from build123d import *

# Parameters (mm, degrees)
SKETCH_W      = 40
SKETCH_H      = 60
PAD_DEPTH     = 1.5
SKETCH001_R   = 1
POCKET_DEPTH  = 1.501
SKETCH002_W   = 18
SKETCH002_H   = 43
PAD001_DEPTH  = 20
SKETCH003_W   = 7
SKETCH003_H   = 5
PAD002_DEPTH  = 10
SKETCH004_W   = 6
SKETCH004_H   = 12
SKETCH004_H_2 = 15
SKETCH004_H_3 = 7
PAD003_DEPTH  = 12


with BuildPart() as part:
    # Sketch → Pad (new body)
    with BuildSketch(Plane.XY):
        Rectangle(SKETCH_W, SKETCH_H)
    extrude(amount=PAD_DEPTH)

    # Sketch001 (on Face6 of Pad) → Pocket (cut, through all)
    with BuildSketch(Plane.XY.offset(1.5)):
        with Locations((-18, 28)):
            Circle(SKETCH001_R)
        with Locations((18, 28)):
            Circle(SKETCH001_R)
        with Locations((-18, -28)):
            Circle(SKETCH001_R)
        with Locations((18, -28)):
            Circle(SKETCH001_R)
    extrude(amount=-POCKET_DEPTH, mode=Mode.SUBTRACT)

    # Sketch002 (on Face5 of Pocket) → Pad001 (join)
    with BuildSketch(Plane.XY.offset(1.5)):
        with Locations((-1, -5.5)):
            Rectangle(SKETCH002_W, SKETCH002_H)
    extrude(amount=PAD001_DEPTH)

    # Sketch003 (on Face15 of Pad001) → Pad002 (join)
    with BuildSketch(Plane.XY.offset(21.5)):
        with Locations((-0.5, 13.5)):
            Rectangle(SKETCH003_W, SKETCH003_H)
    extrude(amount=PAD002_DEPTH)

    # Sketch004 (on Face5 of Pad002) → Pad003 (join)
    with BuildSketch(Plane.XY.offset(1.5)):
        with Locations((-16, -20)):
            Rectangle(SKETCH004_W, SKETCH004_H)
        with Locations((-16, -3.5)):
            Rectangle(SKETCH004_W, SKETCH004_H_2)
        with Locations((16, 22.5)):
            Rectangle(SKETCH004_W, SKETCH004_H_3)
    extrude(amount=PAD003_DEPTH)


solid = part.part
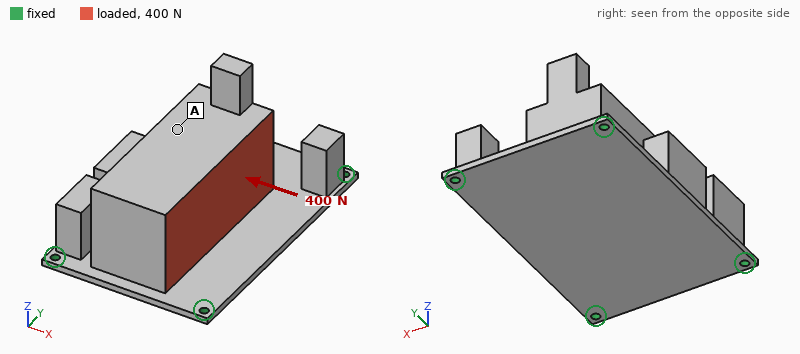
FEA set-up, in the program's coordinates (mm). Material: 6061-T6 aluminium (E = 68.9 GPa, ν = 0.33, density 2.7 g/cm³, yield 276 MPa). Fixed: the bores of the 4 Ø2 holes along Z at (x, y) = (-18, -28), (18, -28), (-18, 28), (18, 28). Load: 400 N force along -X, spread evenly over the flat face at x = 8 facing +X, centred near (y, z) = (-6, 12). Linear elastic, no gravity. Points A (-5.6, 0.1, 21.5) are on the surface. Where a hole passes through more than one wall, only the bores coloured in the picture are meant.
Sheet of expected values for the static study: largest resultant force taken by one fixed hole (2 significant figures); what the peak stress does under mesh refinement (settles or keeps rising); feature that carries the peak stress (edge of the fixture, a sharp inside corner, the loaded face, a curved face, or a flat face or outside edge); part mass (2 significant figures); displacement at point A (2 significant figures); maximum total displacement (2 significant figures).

190 N
keeps rising
edge of the fixture
59 g
67 µm
99 µm
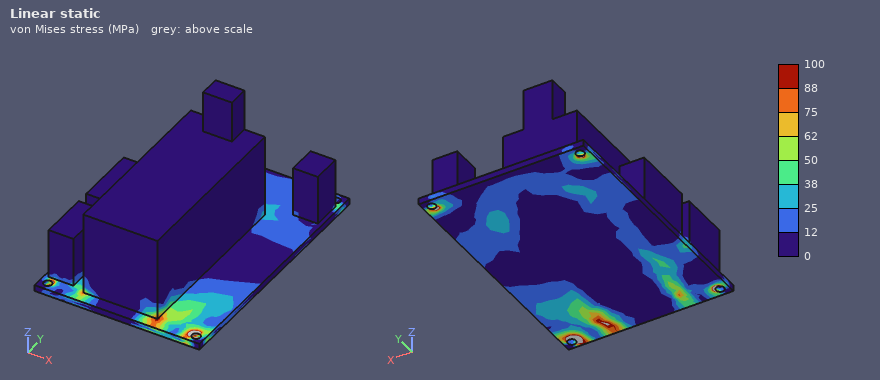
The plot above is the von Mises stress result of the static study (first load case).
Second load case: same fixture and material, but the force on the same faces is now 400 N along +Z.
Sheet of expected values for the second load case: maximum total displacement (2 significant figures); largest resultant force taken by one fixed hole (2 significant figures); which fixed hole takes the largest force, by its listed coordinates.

0.17 mm
200 N
(18, -28)
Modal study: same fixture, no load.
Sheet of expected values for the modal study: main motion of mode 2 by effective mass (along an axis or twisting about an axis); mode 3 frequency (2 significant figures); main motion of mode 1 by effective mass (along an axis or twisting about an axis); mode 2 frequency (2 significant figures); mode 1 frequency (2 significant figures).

along X
2700 Hz
along Z
1900 Hz
1400 Hz
